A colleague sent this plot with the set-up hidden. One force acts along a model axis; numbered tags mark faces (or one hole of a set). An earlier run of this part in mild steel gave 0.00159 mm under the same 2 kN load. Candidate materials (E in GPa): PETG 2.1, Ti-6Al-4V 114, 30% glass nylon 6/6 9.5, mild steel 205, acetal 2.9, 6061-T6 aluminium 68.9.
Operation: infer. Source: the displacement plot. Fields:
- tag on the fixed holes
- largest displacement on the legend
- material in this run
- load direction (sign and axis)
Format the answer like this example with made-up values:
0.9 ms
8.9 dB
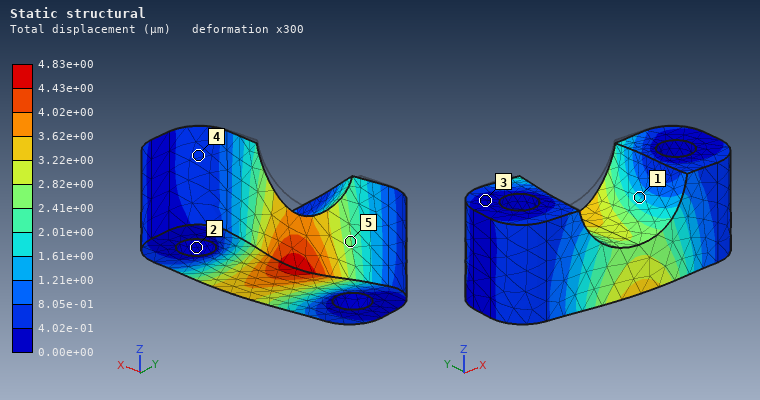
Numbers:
2
4.83e+00 µm
6061-T6 aluminium
-Y
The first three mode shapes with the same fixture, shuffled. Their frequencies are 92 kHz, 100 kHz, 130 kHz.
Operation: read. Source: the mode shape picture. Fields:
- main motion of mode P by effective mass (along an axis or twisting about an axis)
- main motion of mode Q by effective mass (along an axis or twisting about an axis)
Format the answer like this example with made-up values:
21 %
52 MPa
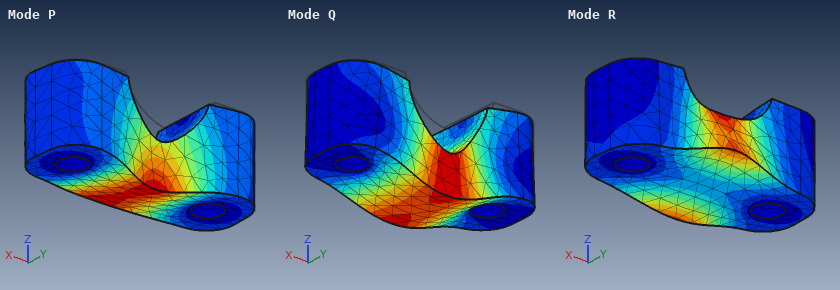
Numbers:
along Y
along Z
